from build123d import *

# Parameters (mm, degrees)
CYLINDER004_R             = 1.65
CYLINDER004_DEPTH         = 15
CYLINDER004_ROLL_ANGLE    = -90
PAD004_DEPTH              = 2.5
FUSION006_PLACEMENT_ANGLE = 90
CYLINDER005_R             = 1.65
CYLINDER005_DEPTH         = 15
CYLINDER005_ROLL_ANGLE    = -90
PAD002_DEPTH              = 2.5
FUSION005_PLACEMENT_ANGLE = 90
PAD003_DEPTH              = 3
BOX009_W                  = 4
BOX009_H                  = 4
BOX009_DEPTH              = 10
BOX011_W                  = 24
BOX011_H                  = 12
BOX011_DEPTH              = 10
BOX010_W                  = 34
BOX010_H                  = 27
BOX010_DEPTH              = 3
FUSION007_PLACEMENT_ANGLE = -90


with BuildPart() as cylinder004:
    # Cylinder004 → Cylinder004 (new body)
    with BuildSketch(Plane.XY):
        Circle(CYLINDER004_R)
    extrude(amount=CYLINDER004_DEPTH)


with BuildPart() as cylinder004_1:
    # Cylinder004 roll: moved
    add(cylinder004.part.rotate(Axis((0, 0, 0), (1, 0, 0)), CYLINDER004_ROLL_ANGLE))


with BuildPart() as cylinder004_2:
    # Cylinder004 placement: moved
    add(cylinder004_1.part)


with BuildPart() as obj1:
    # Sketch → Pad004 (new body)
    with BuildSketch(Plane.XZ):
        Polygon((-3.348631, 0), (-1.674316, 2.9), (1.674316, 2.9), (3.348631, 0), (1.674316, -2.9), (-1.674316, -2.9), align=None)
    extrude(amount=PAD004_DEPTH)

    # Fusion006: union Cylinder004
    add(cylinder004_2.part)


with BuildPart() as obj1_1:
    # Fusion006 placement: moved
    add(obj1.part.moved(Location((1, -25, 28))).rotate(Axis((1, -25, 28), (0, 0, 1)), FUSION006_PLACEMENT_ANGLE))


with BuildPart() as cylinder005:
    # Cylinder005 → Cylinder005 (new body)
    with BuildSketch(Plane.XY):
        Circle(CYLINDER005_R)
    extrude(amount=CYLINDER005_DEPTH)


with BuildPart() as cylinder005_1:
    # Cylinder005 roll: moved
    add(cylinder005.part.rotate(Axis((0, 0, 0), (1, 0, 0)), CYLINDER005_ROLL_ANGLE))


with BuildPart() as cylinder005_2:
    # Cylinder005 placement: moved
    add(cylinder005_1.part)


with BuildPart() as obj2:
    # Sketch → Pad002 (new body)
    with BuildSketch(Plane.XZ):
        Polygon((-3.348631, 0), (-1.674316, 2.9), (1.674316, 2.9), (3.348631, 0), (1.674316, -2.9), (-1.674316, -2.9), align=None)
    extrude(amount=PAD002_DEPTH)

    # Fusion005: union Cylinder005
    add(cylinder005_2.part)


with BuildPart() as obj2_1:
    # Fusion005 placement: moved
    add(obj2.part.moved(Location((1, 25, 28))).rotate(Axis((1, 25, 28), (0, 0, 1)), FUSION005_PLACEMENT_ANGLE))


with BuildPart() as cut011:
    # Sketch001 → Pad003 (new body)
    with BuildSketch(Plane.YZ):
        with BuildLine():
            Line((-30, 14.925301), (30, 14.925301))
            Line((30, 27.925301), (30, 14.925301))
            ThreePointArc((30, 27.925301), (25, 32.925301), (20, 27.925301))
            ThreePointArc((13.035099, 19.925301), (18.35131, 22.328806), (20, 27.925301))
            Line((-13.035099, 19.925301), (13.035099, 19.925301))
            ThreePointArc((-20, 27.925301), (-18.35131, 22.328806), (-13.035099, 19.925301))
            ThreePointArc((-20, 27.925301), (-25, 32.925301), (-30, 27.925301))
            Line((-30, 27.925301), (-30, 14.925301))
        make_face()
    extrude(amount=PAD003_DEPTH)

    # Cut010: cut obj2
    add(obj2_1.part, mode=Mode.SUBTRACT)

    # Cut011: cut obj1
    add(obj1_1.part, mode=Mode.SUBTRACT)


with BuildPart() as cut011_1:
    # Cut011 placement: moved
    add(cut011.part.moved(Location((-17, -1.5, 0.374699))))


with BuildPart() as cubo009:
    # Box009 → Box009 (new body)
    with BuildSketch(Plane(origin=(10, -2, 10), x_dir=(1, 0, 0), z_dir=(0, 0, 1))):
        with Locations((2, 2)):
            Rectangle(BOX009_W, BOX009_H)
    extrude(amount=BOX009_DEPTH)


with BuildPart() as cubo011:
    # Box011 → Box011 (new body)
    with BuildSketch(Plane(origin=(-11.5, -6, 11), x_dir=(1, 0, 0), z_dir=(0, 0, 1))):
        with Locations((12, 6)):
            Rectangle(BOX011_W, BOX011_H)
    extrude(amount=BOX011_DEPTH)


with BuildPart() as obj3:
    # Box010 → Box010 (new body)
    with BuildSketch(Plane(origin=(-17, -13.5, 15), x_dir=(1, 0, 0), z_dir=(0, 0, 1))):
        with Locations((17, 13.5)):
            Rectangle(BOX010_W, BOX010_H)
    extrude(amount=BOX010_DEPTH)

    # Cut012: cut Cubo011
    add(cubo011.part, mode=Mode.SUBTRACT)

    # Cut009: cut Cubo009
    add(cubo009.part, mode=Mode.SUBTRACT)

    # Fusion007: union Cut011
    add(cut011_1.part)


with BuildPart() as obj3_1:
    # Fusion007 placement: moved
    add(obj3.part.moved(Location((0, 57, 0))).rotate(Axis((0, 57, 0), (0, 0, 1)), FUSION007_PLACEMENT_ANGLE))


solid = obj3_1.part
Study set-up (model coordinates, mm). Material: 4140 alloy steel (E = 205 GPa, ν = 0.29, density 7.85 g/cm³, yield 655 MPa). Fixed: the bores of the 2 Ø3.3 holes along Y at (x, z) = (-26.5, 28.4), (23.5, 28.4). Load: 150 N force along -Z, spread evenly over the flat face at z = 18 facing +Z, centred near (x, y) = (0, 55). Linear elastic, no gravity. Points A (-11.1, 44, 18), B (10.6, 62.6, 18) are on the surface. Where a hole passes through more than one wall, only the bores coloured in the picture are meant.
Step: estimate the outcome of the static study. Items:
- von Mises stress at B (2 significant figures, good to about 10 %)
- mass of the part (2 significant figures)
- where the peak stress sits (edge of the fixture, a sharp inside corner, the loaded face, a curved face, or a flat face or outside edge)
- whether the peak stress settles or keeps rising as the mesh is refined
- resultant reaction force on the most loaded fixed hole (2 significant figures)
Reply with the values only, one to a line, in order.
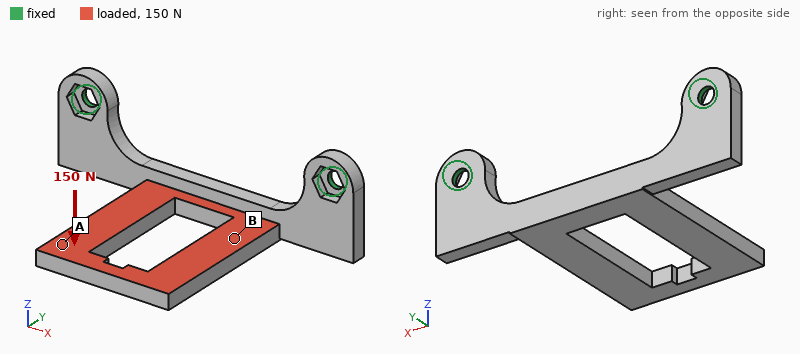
60 MPa
25 g
edge of the fixture
keeps rising
120 N
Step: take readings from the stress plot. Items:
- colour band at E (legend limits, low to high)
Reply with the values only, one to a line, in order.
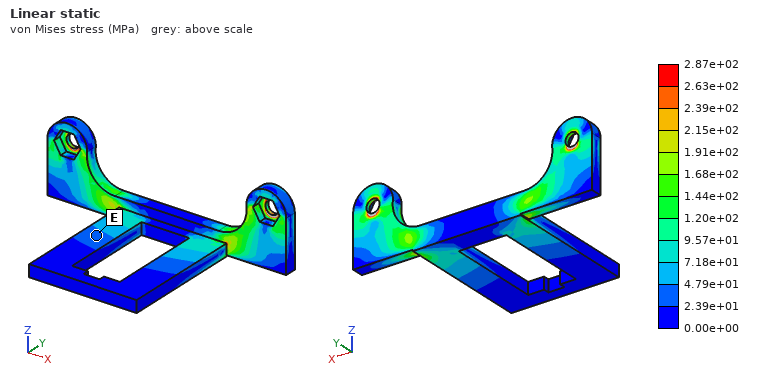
2.39e+01 to 4.79e+01 MPa
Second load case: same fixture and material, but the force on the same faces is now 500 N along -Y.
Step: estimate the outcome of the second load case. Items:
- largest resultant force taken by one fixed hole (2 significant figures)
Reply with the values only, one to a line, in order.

270 N
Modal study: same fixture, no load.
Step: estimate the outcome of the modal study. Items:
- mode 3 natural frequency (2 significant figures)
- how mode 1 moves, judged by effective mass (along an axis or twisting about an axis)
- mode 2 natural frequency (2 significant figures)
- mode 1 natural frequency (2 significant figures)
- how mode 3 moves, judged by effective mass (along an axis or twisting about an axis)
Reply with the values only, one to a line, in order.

3000 Hz
along Z
2800 Hz
990 Hz
along Y
